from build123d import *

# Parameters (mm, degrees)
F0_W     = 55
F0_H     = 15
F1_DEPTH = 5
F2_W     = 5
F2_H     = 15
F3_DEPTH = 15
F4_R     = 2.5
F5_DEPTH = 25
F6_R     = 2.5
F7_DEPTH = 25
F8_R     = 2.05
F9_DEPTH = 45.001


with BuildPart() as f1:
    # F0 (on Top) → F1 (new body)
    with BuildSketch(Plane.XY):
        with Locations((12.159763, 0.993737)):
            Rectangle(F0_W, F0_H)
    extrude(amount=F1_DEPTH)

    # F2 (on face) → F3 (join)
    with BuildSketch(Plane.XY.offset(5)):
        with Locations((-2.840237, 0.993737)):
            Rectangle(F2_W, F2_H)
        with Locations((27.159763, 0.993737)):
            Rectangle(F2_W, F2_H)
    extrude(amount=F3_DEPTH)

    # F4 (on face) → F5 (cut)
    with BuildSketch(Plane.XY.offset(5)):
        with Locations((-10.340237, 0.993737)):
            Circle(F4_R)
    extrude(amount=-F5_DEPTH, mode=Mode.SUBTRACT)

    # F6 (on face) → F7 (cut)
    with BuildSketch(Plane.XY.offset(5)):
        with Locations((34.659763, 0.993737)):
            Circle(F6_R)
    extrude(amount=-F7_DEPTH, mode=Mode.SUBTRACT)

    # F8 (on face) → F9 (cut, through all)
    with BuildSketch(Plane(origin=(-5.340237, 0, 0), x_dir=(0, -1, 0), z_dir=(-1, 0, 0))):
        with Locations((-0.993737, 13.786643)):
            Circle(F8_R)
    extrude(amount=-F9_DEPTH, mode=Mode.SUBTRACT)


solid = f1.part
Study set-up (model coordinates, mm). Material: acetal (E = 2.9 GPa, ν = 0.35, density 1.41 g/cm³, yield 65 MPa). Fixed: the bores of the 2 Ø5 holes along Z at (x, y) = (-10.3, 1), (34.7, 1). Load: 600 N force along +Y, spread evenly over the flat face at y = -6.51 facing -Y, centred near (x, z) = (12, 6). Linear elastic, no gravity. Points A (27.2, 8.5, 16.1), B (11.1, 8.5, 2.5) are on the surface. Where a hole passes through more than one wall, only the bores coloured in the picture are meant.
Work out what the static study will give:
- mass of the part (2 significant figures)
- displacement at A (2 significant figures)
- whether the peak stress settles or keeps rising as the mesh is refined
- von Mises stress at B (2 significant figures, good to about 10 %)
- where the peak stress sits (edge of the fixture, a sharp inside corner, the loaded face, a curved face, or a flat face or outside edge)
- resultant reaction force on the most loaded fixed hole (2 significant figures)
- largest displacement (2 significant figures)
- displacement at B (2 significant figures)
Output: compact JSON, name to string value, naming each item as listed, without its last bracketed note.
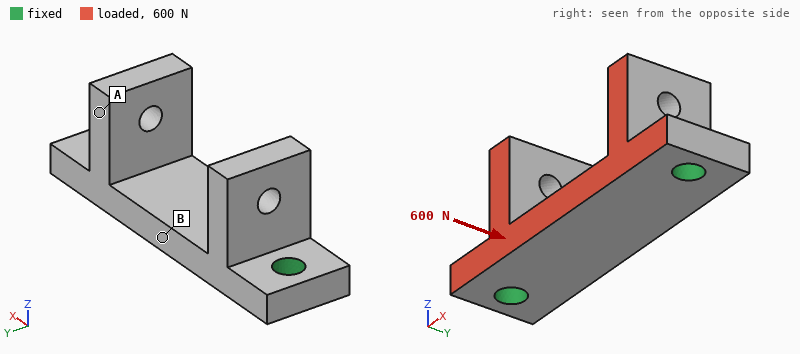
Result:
{"mass of the part": "8.5 g", "displacement at A": "0.18 mm", "whether the peak stress settles or keeps rising as the mesh is refined": "keeps rising", "von Mises stress at B": "6.0 MPa", "where the peak stress sits": "edge of the fixture", "resultant reaction force on the most loaded fixed hole": "300 N", "largest displacement": "0.22 mm", "displacement at B": "0.095 mm"}
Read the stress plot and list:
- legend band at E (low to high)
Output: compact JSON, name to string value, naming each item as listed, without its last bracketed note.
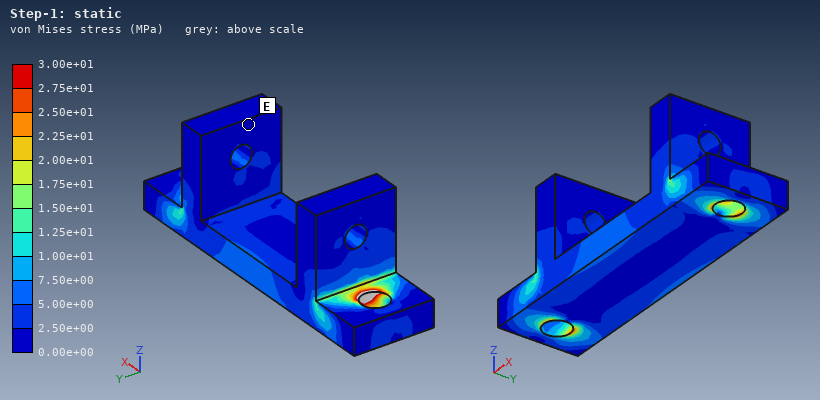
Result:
{"legend band at E": "0.00e+00 to 2.50e+00 MPa"}
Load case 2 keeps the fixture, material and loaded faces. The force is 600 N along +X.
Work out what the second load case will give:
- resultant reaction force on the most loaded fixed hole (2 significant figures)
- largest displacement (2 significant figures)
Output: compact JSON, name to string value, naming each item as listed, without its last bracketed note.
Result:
{"resultant reaction force on the most loaded fixed hole": "310 N", "largest displacement": "0.33 mm"}
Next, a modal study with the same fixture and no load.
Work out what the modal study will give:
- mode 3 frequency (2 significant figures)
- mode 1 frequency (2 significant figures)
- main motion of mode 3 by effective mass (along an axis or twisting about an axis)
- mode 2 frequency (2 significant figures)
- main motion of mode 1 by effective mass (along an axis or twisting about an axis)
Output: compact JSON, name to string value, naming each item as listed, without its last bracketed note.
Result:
{"mode 3 frequency": "3400 Hz", "mode 1 frequency": "2500 Hz", "main motion of mode 3 by effective mass": "along X", "mode 2 frequency": "3300 Hz", "main motion of mode 1 by effective mass": "along Z"}
